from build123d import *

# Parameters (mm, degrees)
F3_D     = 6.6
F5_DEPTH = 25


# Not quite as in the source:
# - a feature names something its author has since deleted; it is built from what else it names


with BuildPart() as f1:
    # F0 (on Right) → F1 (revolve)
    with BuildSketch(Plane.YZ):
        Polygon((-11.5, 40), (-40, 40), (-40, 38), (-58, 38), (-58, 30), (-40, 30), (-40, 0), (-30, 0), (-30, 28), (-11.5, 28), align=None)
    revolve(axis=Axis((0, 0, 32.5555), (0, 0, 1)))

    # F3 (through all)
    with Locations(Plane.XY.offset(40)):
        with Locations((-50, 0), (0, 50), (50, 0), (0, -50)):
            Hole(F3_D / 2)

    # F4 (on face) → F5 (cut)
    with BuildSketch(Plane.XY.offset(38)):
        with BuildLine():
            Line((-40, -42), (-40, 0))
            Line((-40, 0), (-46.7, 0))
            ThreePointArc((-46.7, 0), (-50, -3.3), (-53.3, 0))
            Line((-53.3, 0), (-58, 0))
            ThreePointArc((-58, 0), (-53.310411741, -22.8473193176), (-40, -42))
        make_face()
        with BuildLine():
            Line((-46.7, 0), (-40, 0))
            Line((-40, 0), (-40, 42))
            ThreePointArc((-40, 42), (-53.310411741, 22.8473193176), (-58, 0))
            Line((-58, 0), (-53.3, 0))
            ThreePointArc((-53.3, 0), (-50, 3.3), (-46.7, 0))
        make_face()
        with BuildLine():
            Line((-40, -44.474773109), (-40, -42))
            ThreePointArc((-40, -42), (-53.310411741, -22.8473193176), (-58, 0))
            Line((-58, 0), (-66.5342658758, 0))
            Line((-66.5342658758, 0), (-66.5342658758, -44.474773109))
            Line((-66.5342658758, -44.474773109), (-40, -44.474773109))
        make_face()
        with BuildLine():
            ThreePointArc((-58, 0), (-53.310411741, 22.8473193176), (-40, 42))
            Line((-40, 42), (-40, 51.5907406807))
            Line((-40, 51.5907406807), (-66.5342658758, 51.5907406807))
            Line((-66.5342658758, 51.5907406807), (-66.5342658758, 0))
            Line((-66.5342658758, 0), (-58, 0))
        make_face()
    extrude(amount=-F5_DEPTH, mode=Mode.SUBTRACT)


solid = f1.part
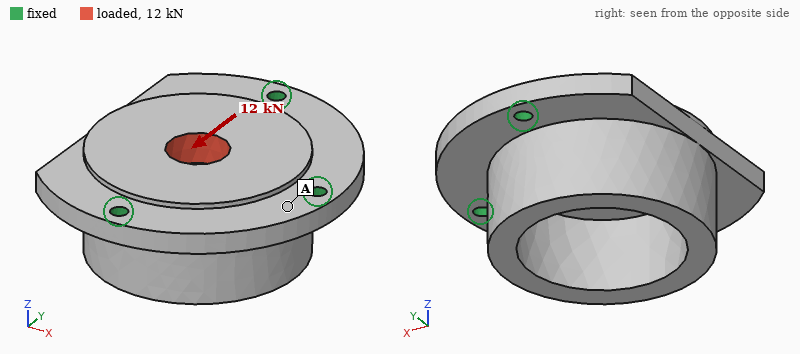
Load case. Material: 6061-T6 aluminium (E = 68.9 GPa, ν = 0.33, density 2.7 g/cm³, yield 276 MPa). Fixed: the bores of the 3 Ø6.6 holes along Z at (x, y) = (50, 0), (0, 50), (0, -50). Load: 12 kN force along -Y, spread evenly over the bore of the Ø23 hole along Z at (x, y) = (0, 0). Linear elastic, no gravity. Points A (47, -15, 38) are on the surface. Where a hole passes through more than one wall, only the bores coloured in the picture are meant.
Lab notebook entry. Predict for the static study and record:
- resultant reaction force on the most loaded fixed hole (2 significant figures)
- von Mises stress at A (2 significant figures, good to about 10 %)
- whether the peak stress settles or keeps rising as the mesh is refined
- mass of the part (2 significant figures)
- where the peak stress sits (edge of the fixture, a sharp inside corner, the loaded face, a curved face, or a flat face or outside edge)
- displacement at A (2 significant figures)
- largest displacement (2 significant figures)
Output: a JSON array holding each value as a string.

["5.0 kN", "7.4 MPa", "keeps rising", "410 g", "edge of the fixture", "2.6 µm", "13 µm"]
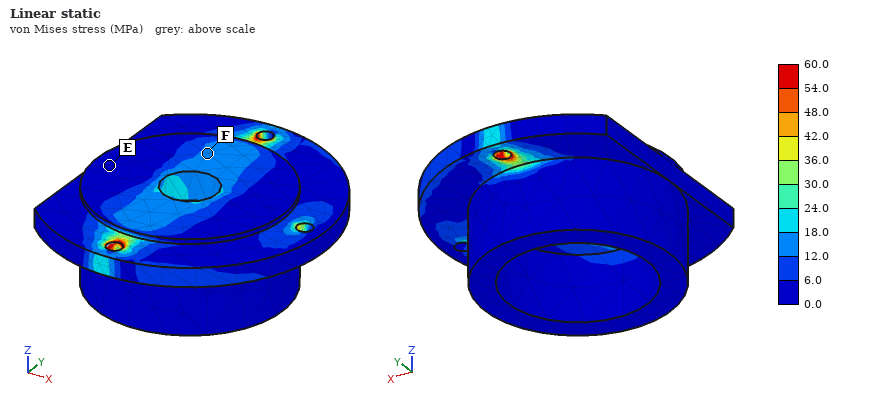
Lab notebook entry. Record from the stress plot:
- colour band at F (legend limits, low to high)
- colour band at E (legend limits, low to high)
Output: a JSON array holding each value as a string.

["12.0 to 18.0 MPa", "0.0 to 6.0 MPa"]
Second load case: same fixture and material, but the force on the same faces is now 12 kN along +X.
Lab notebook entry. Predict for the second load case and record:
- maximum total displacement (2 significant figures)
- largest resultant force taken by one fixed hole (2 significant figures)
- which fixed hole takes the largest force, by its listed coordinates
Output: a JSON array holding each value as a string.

["17 µm", "5.0 kN", "(50, 0)"]
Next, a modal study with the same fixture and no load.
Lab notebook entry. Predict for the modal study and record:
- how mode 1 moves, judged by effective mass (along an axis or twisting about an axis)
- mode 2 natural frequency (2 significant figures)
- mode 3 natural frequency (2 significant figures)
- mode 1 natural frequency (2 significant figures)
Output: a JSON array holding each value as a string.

["along Z", "6700 Hz", "6900 Hz", "2800 Hz"]
